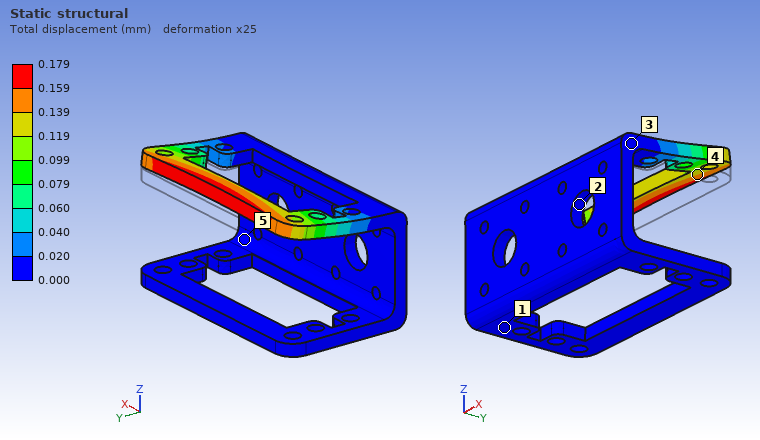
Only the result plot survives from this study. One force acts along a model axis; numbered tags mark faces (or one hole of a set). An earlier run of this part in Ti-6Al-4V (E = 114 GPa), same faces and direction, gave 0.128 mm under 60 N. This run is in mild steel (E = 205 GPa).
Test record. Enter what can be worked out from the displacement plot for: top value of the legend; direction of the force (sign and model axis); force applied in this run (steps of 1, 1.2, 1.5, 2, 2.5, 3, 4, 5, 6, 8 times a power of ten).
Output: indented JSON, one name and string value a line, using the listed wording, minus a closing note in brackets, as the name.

{
  "top value of the legend": "0.179 mm",
  "direction of the force": "+Z",
  "force applied in this run": "150 N"
}
